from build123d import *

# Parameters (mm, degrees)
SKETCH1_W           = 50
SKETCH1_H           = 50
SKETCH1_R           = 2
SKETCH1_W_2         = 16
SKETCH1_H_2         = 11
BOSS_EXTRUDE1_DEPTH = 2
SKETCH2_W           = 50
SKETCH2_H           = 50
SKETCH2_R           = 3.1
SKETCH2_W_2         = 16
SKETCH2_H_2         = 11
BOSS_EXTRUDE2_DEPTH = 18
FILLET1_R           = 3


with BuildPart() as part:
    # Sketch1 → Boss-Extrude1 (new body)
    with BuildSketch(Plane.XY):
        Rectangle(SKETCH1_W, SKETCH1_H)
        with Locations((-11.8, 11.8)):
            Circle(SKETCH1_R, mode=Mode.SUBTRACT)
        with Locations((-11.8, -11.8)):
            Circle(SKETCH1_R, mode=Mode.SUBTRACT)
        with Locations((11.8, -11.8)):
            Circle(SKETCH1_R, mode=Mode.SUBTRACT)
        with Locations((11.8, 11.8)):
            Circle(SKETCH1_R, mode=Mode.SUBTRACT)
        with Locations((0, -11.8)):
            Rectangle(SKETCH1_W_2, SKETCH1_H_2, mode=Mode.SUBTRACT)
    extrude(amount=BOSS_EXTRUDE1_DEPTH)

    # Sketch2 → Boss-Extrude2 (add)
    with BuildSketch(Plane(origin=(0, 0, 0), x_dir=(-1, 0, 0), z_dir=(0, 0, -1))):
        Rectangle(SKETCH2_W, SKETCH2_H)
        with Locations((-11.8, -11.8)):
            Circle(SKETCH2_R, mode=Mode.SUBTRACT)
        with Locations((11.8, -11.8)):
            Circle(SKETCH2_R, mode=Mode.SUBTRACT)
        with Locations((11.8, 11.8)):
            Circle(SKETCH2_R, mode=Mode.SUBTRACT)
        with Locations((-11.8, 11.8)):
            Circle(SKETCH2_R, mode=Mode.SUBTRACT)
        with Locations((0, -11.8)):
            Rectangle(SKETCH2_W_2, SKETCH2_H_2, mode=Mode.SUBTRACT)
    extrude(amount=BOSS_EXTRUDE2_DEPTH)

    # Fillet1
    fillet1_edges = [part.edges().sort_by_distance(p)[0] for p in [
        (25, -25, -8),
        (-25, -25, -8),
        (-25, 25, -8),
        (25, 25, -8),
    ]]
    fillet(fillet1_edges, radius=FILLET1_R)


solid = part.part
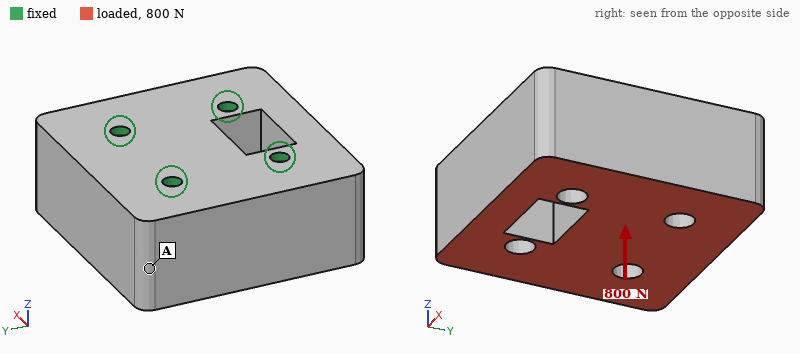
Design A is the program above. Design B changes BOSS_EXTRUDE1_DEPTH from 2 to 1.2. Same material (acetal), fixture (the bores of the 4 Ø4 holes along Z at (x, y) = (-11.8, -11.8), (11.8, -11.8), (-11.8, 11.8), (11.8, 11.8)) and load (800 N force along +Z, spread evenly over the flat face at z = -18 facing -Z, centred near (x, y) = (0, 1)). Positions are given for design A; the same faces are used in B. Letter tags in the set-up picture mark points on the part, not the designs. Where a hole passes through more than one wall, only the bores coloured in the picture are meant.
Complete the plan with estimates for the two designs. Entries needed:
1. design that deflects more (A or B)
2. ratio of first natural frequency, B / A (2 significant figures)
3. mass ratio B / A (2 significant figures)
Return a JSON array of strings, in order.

["B", "0.82", "0.96"]
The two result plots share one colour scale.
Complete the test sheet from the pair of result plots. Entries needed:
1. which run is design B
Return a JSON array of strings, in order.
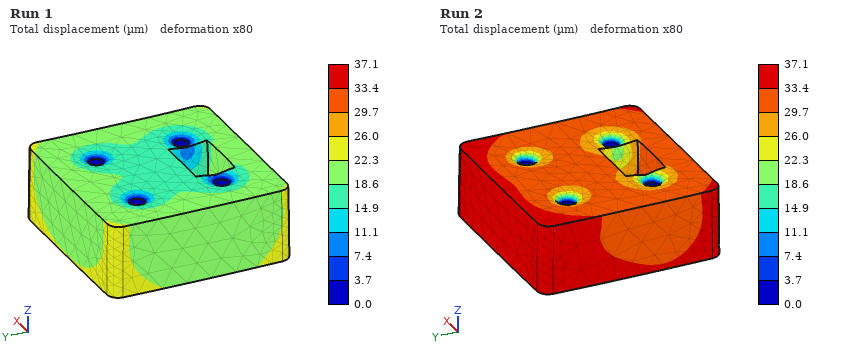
["Run 2"]
